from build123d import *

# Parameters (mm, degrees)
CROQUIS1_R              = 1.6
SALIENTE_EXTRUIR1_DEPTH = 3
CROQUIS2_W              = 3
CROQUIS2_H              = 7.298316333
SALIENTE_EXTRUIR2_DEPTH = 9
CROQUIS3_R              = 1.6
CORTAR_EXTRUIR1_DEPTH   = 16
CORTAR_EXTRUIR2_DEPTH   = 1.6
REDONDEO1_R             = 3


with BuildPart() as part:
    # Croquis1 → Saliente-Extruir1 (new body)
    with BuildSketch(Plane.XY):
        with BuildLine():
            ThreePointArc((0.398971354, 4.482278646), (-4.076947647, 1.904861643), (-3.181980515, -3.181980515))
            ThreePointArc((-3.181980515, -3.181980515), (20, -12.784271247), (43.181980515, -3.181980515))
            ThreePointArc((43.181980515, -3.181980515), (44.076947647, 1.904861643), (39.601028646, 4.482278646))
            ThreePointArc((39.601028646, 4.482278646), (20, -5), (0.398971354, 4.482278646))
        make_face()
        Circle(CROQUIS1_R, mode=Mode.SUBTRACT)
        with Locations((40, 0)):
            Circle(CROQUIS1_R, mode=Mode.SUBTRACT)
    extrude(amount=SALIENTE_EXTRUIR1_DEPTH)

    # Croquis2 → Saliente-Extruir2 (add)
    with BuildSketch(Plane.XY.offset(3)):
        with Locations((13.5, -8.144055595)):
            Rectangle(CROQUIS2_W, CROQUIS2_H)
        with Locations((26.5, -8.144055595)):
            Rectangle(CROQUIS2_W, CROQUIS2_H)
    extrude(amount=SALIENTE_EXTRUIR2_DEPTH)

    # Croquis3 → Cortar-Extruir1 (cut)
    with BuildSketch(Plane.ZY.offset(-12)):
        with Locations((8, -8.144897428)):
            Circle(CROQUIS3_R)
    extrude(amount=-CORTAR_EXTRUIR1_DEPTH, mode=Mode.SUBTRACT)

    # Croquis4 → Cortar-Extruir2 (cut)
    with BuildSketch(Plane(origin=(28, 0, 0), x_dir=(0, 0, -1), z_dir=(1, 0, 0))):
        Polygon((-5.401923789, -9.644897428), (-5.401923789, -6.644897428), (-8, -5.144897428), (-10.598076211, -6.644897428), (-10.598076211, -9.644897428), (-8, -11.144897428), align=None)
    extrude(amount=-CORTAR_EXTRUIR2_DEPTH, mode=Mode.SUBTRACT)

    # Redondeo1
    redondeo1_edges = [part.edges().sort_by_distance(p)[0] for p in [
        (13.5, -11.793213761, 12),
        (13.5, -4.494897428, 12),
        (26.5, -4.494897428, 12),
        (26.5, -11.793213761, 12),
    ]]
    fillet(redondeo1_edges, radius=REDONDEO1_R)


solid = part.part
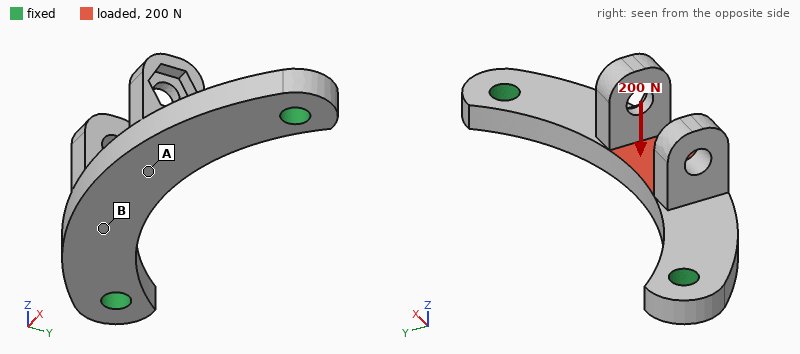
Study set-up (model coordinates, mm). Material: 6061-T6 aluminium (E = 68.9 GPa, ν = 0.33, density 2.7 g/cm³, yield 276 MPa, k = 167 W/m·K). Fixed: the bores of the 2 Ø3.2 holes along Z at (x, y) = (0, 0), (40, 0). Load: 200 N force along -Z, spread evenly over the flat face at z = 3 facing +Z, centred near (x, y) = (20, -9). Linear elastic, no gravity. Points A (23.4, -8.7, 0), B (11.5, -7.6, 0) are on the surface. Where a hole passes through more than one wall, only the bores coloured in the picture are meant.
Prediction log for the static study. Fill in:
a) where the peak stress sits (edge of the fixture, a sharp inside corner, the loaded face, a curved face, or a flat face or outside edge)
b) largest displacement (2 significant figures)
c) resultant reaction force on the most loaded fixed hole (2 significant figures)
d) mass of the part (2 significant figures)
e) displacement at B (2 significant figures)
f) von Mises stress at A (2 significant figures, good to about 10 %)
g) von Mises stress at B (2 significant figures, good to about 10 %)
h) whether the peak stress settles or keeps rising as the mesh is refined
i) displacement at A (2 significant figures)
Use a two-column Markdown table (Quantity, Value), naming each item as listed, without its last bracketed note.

| Quantity | Value |
|---|---|
| where the peak stress sits | edge of the fixture |
| largest displacement | 100 µm |
| resultant reaction force on the most loaded fixed hole | 100 N |
| mass of the part | 4.0 g |
| displacement at B | 54 µm |
| von Mises stress at A | 58 MPa |
| von Mises stress at B | 22 MPa |
| whether the peak stress settles or keeps rising as the mesh is refined | keeps rising |
| displacement at A | 75 µm |
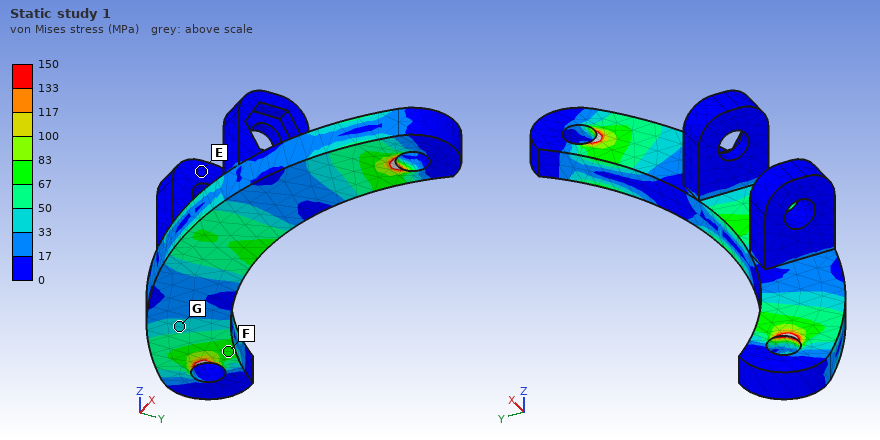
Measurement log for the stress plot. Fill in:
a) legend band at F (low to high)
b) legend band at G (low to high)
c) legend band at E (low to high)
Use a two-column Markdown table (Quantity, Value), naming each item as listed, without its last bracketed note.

| Quantity | Value |
|---|---|
| legend band at F | 67 to 83 MPa |
| legend band at G | 33 to 50 MPa |
| legend band at E | 0 to 17 MPa |
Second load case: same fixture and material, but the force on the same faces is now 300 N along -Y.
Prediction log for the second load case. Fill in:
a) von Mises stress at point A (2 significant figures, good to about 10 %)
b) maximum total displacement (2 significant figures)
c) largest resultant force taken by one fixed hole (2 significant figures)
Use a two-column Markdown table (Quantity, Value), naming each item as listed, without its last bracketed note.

| Quantity | Value |
|---|---|
| von Mises stress at point A | 9.9 MPa |
| maximum total displacement | 33 µm |
| largest resultant force taken by one fixed hole | 250 N |
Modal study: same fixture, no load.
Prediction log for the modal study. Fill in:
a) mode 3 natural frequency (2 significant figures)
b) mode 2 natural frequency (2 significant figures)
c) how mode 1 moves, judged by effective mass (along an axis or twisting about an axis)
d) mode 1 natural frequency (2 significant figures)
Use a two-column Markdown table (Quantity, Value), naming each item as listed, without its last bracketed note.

| Quantity | Value |
|---|---|
| mode 3 natural frequency | 15 kHz |
| mode 2 natural frequency | 12 kHz |
| how mode 1 moves, judged by effective mass | along Z |
| mode 1 natural frequency | 5700 Hz |
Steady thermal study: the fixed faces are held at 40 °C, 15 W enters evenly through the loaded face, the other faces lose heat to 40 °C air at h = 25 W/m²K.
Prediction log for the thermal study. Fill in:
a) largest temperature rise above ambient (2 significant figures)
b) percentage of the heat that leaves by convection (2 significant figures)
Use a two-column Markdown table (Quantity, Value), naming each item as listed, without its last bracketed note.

| Quantity | Value |
|---|---|
| largest temperature rise above ambient | 36 K |
| percentage of the heat that leaves by convection | 4.4 % |
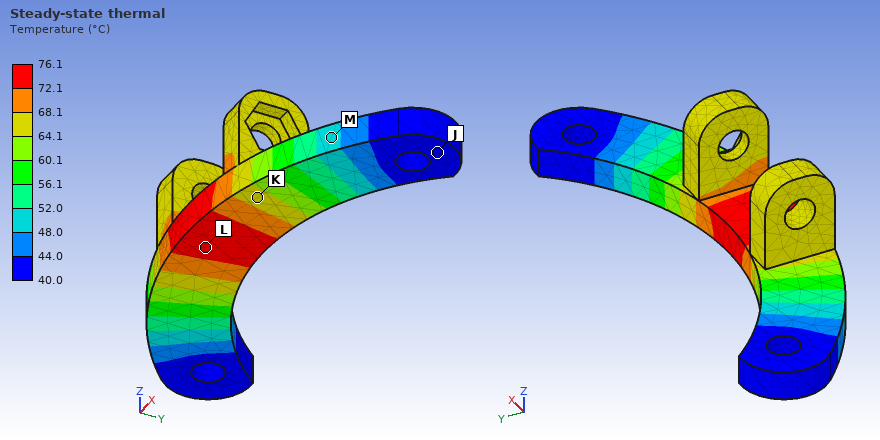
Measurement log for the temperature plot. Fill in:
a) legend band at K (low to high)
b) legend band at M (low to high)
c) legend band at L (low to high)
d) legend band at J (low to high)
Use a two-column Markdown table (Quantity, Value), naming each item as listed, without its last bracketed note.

| Quantity | Value |
|---|---|
| legend band at K | 64.1 to 68.1 °C |
| legend band at M | 48.0 to 52.0 °C |
| legend band at L | 72.1 to 76.1 °C |
| legend band at J | 40.0 to 44.0 °C |
